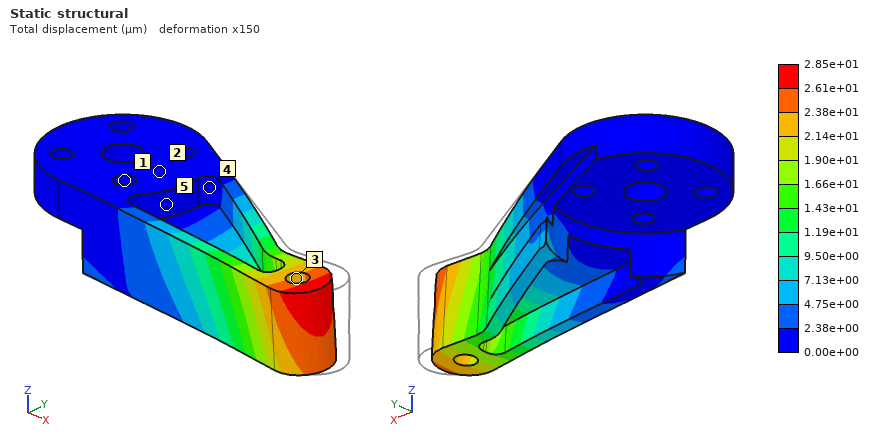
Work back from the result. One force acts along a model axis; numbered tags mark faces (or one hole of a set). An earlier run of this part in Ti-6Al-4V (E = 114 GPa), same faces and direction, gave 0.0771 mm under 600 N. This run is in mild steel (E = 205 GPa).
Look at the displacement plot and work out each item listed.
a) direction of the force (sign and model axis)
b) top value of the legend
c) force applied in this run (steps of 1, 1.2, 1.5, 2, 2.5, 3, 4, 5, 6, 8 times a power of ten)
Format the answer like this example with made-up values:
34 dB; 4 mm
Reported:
-Y; 2.85e+01 µm; 400 N
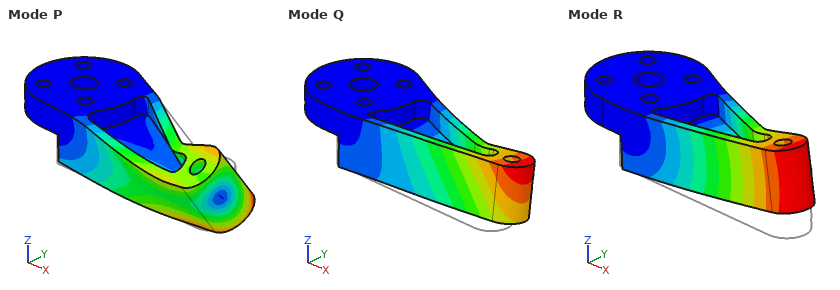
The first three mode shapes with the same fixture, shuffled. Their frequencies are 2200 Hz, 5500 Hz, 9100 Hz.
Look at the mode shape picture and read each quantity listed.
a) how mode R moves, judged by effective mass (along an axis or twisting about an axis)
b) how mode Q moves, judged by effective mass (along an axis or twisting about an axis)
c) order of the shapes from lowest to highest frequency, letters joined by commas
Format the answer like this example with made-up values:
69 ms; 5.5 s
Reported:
along Z; along Y; R, Q, P
